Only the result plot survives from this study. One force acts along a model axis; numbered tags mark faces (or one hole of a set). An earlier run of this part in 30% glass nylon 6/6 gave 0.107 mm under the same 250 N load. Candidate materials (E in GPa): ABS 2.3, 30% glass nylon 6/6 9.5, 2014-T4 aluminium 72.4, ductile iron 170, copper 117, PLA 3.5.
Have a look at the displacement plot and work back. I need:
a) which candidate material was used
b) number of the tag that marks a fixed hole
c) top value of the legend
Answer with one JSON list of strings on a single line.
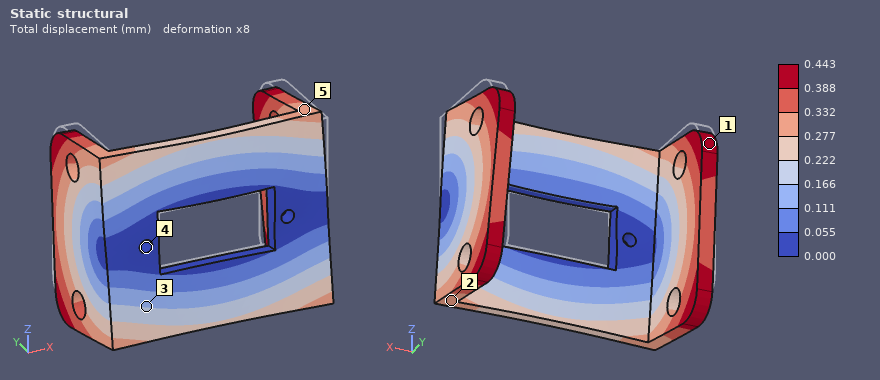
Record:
["ABS", "4", "0.443 mm"]
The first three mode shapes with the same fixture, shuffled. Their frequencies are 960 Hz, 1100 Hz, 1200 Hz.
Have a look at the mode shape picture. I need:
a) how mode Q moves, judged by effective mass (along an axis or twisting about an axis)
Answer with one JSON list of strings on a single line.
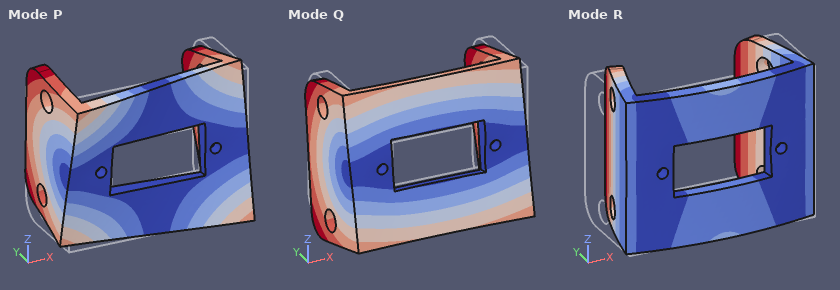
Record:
["along Z"]
